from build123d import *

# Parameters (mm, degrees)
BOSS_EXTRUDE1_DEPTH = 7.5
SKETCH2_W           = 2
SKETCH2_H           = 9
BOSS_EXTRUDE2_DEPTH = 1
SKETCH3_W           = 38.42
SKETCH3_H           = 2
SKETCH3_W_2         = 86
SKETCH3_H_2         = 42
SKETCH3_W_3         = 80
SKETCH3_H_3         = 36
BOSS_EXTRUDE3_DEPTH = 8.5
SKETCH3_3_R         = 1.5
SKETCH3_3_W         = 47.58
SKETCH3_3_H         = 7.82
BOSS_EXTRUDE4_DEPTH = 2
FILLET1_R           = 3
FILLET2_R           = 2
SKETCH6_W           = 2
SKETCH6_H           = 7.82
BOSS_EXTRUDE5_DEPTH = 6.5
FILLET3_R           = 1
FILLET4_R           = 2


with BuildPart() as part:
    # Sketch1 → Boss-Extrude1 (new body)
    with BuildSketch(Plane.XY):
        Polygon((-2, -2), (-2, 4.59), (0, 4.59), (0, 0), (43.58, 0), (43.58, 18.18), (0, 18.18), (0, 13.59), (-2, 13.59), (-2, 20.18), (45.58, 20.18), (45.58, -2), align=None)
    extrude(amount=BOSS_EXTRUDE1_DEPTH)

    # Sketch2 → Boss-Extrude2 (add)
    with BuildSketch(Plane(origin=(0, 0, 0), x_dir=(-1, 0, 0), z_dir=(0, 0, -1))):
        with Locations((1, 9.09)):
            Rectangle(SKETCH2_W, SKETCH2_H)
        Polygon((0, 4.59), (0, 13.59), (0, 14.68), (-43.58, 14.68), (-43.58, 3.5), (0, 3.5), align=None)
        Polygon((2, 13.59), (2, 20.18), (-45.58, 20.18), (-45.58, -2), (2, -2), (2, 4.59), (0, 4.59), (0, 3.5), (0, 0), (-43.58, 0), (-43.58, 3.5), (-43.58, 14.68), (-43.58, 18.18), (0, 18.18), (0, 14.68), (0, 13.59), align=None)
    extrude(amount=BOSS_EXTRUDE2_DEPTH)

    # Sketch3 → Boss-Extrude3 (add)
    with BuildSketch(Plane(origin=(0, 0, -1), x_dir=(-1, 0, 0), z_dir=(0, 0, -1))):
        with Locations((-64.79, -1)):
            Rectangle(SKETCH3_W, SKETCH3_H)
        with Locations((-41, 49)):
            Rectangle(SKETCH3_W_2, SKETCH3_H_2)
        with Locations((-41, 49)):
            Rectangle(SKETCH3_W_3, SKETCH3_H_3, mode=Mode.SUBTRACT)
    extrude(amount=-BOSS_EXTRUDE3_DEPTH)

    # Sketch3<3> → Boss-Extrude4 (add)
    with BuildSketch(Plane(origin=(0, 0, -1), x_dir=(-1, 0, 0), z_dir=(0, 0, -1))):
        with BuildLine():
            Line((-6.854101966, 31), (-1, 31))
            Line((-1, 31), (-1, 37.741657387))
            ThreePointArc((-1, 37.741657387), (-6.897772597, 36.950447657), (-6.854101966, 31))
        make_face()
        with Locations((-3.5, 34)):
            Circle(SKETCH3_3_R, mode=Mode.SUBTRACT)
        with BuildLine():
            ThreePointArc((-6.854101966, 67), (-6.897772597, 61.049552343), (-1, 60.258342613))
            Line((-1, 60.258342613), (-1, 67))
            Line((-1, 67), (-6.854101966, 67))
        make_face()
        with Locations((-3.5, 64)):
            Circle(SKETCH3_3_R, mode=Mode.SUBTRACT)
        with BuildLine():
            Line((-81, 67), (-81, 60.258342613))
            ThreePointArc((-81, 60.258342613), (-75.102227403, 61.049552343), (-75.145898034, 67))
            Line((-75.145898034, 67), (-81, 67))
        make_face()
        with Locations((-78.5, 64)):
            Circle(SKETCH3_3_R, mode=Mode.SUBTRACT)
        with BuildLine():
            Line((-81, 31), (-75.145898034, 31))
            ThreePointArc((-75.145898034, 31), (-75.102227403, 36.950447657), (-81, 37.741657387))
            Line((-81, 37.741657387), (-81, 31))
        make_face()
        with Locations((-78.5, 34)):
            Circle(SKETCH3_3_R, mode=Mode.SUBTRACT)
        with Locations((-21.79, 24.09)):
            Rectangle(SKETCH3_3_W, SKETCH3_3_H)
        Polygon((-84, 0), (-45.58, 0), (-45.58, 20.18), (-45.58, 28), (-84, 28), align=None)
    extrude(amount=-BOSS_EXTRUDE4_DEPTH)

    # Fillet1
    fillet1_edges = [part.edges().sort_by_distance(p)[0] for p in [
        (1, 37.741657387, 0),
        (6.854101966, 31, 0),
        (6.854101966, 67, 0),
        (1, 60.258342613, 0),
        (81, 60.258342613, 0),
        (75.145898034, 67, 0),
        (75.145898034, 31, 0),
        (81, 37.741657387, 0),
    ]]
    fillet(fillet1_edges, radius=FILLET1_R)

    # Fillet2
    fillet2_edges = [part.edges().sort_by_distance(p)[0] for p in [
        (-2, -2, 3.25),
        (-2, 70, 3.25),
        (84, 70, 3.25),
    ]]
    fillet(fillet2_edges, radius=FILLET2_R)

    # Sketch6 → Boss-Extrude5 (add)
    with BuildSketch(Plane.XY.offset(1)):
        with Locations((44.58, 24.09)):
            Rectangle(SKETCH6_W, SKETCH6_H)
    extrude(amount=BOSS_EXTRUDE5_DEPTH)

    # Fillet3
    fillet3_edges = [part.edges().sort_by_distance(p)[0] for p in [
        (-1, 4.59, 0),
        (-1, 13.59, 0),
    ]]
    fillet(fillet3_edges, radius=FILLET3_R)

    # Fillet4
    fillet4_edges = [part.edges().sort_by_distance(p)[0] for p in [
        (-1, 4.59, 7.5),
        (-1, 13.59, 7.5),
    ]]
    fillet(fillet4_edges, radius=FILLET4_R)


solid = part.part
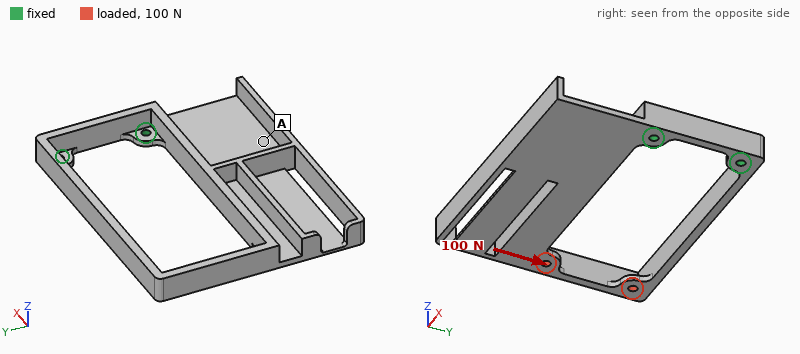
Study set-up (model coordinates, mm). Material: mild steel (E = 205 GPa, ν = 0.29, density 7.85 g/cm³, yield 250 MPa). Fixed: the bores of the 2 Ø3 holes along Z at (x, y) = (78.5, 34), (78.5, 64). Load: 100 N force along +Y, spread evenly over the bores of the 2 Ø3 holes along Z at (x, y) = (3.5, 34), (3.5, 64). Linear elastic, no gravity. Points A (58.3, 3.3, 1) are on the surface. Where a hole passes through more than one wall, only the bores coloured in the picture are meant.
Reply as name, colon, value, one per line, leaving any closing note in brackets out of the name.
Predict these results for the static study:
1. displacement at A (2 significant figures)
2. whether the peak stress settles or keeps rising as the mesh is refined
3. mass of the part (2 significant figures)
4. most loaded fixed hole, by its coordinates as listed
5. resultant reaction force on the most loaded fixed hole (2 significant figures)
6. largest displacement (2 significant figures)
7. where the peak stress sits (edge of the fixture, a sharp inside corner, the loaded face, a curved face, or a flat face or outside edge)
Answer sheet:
displacement at A: 0.057 mm
whether the peak stress settles or keeps rising as the mesh is refined: keeps rising
mass of the part: 100 g
most loaded fixed hole, by its coordinates as listed: (78.5, 34)
resultant reaction force on the most loaded fixed hole: 260 N
largest displacement: 0.15 mm
where the peak stress sits: edge of the fixture
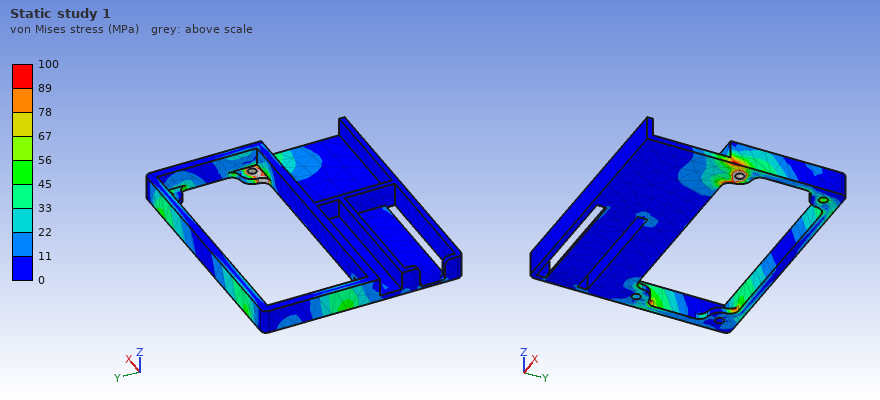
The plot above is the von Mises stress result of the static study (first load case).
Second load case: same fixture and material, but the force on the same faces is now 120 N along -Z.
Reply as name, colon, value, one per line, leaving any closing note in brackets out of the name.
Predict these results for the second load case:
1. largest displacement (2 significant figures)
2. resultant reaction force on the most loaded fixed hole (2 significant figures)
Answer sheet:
largest displacement: 0.52 mm
resultant reaction force on the most loaded fixed hole: 100 N
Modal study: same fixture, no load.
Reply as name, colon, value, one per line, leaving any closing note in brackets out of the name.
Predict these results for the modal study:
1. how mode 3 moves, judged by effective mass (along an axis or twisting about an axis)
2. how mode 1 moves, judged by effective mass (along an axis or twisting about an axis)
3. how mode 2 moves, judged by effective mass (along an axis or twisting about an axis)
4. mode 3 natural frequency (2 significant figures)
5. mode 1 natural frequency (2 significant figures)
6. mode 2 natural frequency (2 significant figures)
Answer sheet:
how mode 3 moves, judged by effective mass: along Y
how mode 1 moves, judged by effective mass: along Z
how mode 2 moves, judged by effective mass: along Y
mode 3 natural frequency: 750 Hz
mode 1 natural frequency: 380 Hz
mode 2 natural frequency: 640 Hz
